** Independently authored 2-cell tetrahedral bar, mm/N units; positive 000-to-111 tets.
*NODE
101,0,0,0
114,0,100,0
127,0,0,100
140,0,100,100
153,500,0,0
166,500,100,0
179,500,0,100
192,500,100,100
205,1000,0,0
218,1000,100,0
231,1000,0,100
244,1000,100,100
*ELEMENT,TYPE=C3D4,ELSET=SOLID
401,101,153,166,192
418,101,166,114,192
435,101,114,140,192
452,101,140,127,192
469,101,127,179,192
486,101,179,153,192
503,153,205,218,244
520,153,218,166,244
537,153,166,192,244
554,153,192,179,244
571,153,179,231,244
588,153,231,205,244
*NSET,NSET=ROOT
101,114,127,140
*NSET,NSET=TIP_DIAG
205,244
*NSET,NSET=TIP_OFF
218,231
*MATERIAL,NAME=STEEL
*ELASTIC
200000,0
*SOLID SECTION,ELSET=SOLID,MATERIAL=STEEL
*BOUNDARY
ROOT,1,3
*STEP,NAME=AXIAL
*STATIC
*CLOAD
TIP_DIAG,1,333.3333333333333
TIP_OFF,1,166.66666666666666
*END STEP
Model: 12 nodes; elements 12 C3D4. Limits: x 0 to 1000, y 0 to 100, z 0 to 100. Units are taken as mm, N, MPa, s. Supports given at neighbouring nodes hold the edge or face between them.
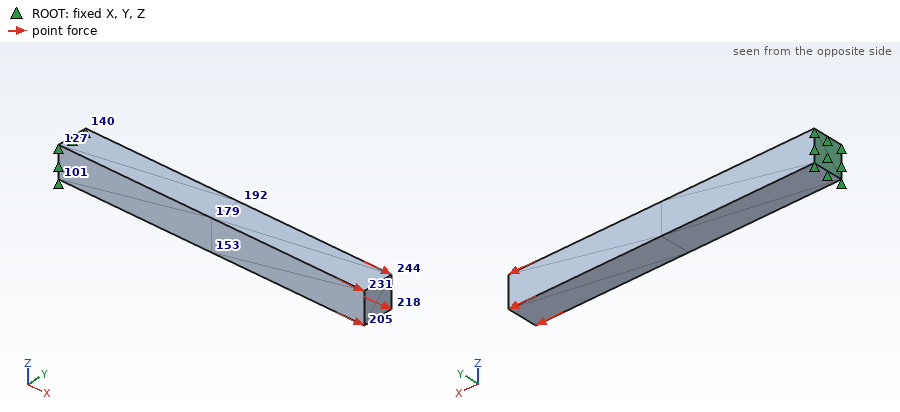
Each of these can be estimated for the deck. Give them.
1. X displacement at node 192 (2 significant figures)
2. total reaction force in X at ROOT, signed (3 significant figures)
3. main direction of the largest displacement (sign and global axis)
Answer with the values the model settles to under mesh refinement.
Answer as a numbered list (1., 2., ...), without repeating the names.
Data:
1. 2.5e-04 mm
2. -1000 N
3. +X
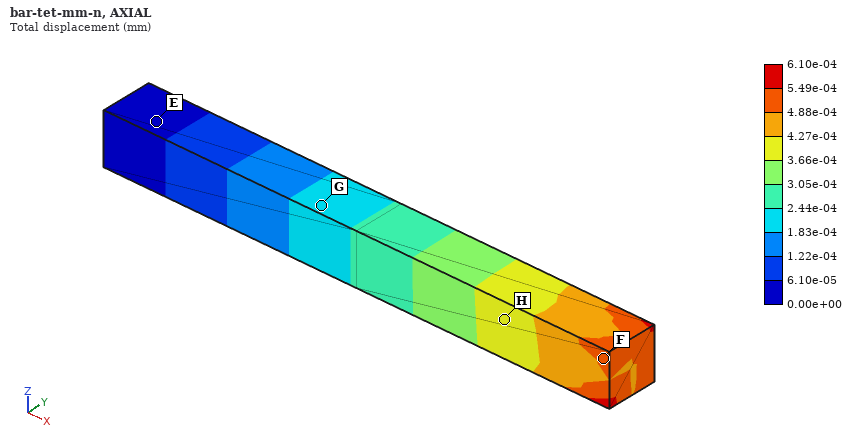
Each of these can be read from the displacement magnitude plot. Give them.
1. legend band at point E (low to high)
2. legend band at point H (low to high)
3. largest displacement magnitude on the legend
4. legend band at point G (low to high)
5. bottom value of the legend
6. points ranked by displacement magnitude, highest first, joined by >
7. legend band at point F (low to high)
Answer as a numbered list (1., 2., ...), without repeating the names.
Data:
1. 0.00e+00 to 6.10e-05 mm
2. 3.66e-04 to 4.27e-04 mm
3. 6.10e-04 mm
4. 1.83e-04 to 2.44e-04 mm
5. 0.00e+00 mm
6. F > H > G > E
7. 4.88e-04 to 5.49e-04 mm
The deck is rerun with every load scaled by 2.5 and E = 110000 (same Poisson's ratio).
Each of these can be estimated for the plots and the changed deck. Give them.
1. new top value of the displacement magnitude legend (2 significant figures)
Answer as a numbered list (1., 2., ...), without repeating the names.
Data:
1. 0.0028 mm
